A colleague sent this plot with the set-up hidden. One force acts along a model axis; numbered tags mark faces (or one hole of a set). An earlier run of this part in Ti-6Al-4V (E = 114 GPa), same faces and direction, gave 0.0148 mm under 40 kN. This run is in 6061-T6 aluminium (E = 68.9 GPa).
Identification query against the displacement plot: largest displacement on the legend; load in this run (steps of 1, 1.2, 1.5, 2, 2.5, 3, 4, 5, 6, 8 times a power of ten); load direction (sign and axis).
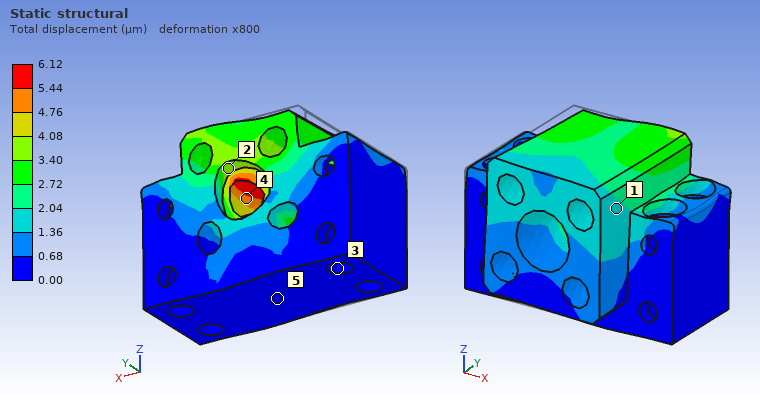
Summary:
6.12 µm
10 kN
+X
